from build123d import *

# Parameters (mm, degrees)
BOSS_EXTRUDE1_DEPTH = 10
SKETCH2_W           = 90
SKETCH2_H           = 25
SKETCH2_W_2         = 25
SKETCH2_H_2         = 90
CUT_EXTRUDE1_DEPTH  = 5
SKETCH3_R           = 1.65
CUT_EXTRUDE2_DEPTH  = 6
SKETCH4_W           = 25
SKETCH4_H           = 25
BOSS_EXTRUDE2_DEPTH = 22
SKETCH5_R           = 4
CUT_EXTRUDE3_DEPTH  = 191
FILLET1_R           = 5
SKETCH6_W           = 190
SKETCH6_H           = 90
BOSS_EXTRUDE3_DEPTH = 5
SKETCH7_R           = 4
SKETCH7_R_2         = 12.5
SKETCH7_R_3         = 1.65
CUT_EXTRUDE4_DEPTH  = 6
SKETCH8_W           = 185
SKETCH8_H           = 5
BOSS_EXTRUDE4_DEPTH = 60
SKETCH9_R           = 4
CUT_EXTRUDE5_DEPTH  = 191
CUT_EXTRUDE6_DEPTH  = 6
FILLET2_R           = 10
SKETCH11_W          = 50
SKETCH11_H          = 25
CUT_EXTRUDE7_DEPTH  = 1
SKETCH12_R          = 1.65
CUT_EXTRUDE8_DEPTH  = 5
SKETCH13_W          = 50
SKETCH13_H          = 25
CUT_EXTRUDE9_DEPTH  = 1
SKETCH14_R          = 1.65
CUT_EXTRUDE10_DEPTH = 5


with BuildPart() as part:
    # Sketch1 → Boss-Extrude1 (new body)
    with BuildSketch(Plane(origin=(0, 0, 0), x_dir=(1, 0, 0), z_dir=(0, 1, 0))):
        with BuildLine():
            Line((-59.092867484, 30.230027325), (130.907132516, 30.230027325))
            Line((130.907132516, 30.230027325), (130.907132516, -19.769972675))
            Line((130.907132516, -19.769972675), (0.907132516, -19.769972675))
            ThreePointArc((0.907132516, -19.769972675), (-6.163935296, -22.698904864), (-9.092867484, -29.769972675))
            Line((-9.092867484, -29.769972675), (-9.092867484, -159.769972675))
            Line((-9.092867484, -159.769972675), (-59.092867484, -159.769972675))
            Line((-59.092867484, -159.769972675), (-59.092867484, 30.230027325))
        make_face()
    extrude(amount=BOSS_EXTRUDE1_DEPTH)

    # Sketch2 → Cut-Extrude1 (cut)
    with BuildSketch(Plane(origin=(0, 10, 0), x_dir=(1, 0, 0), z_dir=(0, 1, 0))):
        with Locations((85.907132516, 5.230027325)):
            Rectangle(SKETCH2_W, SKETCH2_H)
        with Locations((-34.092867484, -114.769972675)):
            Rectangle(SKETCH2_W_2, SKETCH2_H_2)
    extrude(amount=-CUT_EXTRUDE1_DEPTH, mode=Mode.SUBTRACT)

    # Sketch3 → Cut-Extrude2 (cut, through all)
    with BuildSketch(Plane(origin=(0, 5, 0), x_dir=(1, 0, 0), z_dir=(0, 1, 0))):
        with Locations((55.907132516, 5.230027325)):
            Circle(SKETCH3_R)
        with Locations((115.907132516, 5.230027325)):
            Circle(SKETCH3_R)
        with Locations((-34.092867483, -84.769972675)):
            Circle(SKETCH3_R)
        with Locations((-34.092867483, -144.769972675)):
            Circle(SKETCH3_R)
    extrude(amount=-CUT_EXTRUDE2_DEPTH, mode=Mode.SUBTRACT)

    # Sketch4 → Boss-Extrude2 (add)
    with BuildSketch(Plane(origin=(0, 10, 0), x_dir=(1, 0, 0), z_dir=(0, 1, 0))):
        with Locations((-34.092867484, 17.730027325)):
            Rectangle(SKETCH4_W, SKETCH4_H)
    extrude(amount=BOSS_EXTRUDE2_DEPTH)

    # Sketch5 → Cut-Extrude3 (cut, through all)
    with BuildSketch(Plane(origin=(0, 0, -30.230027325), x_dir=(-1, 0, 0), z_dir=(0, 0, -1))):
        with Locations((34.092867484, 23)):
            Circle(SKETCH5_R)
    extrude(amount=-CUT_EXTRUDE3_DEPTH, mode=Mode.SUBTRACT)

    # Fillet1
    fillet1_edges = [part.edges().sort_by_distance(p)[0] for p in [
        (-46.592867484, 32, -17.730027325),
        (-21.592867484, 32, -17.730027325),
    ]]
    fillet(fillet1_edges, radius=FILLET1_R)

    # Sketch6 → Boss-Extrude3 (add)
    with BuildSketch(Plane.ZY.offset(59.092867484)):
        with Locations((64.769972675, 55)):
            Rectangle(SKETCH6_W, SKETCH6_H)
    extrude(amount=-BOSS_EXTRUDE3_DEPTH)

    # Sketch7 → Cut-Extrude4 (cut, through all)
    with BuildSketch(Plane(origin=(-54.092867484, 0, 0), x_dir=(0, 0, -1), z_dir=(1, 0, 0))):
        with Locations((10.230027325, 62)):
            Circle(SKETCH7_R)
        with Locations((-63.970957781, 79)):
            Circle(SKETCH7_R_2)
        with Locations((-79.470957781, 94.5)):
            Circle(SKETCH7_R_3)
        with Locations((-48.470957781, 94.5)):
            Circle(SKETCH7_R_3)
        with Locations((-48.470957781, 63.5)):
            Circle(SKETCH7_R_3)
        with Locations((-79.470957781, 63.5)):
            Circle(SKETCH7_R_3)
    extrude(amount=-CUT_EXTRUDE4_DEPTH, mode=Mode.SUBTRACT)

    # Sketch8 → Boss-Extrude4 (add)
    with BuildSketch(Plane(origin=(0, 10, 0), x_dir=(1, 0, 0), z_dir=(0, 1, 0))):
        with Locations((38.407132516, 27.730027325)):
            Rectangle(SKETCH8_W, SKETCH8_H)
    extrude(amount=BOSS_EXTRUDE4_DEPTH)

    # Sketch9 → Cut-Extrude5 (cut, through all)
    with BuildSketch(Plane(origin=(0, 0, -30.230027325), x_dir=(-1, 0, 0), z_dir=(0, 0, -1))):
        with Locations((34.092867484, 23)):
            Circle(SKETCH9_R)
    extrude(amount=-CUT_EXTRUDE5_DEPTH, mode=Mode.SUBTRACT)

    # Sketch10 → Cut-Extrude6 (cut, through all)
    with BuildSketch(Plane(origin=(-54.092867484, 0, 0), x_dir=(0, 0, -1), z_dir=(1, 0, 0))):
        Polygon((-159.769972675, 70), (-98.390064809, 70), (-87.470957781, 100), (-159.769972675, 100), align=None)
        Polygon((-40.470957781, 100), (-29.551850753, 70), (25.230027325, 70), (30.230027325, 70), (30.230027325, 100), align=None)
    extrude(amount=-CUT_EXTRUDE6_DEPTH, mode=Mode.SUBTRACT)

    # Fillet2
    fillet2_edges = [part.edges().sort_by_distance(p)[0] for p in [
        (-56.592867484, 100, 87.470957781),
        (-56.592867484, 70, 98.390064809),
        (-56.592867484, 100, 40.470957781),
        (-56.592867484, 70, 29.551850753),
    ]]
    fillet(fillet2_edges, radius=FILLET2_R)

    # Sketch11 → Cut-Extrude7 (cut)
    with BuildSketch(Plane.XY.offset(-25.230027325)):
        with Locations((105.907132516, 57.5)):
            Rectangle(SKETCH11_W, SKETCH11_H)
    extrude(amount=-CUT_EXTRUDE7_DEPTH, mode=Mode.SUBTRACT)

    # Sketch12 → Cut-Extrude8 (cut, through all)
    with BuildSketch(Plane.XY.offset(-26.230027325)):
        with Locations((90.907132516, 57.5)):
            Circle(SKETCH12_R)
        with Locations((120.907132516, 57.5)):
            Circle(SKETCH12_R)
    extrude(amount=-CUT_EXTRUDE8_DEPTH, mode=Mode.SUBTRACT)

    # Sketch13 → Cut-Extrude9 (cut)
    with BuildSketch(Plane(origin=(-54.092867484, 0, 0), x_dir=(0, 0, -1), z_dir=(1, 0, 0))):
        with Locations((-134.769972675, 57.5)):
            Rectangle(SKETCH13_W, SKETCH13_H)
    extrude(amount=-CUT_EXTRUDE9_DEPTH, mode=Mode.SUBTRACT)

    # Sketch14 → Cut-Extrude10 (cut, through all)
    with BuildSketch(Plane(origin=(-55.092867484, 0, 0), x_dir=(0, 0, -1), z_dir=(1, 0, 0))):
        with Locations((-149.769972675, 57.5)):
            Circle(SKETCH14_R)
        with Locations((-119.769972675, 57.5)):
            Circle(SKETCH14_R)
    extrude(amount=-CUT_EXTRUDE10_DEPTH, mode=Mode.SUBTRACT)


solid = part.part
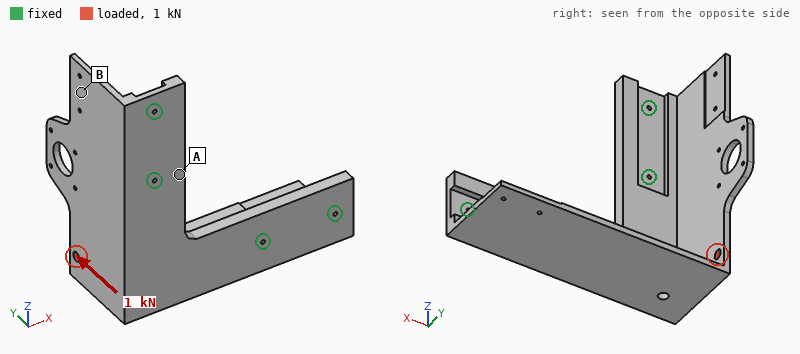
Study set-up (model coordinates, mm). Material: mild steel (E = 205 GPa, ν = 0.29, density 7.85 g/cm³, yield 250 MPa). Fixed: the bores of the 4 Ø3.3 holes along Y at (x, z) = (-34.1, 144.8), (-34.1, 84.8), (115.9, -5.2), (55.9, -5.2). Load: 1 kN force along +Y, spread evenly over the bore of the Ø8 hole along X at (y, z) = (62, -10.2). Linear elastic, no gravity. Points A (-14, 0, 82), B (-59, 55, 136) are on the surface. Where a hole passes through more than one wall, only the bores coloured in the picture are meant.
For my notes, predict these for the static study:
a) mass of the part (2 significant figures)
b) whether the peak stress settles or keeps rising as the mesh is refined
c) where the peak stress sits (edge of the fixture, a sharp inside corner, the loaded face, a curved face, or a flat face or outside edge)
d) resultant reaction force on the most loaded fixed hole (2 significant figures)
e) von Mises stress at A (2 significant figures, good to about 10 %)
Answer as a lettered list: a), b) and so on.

a) 2.1 kg
b) keeps rising
c) edge of the fixture
d) 1.5 kN
e) 17 MPa
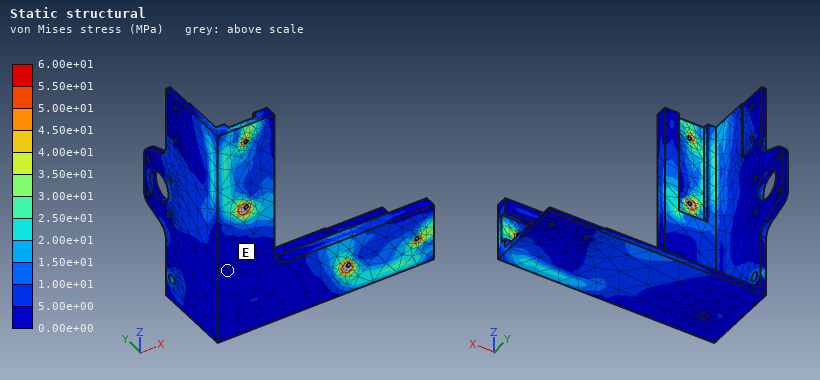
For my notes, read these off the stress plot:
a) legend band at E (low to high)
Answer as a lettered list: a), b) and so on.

a) 0.00e+00 to 5.00e+00 MPa
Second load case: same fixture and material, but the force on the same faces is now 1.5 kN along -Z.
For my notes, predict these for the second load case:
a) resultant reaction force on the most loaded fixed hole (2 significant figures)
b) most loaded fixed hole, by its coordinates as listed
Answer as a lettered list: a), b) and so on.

a) 1.2 kN
b) (-34.1, 144.8)
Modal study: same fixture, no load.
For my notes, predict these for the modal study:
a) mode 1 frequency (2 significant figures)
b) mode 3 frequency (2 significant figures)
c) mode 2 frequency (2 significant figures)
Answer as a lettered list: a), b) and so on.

a) 600 Hz
b) 880 Hz
c) 720 Hz
